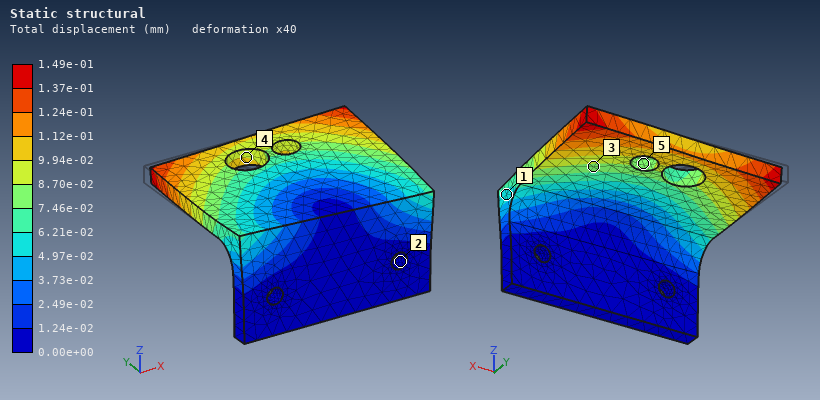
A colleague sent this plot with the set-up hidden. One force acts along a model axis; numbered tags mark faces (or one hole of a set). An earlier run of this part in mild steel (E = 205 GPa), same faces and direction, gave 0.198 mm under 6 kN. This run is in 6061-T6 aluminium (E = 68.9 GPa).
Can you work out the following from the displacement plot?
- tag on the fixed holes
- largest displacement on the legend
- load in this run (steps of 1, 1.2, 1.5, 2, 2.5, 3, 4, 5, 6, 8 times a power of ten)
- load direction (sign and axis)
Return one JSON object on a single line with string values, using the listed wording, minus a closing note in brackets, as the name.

{"tag on the fixed holes": "2", "largest displacement on the legend": "1.49e-01 mm", "load in this run": "1.5 kN", "load direction": "+X"}
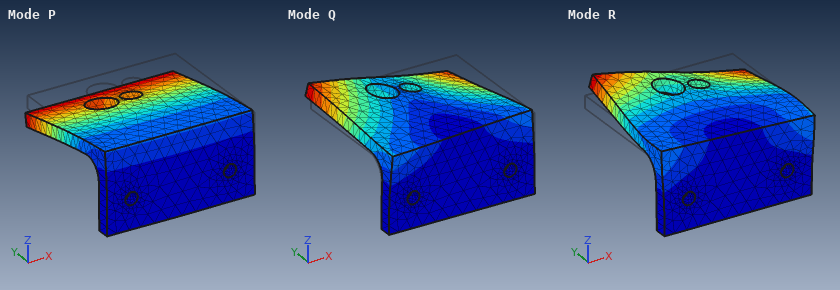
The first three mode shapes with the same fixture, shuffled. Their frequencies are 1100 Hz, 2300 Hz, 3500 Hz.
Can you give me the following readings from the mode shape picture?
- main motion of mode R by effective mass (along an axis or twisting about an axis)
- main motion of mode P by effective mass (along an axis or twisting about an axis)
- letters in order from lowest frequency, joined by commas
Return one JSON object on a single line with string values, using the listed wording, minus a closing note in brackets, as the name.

{"main motion of mode R by effective mass": "along X", "main motion of mode P by effective mass": "along Z", "letters in order from lowest frequency, joined by commas": "P, Q, R"}
